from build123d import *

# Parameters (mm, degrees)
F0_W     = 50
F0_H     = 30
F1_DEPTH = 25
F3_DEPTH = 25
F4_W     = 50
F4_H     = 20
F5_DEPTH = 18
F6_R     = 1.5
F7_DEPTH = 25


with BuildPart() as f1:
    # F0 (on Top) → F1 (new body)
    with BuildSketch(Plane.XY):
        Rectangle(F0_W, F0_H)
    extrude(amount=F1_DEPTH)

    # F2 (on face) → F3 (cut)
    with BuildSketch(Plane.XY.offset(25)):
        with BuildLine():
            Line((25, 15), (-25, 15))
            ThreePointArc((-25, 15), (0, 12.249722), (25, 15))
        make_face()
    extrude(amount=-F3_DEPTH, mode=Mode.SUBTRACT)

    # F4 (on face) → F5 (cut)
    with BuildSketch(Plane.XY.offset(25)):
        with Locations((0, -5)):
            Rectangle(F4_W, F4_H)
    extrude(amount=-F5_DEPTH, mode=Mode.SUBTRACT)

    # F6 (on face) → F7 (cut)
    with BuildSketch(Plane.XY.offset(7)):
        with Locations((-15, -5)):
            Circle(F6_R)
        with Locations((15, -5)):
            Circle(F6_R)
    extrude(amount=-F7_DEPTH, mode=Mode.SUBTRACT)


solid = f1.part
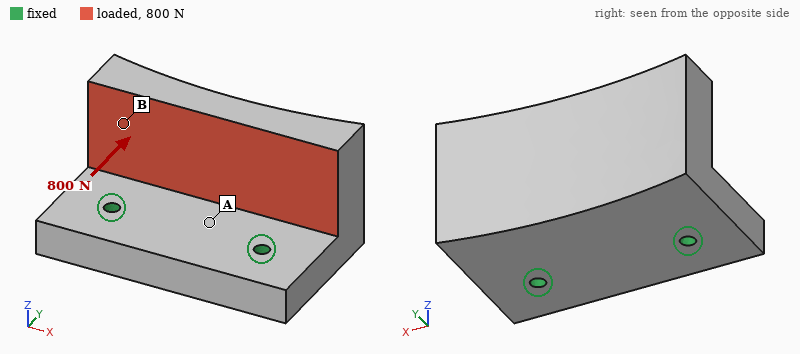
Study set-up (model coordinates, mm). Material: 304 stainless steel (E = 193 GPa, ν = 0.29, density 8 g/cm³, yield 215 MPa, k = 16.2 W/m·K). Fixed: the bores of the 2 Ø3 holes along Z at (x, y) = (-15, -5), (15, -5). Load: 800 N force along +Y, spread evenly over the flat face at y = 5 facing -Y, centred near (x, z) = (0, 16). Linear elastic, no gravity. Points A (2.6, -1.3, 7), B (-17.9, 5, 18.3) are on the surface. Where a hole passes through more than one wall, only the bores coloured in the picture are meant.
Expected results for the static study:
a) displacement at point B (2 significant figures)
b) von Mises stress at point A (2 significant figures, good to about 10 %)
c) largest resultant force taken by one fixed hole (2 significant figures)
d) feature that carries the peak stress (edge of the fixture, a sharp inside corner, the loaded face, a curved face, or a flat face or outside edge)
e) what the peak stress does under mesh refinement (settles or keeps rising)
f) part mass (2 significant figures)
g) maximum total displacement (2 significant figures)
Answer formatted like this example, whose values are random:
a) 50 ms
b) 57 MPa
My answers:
a) 10 µm
b) 16 MPa
c) 400 N
d) edge of the fixture
e) keeps rising
f) 140 g
g) 17 µm
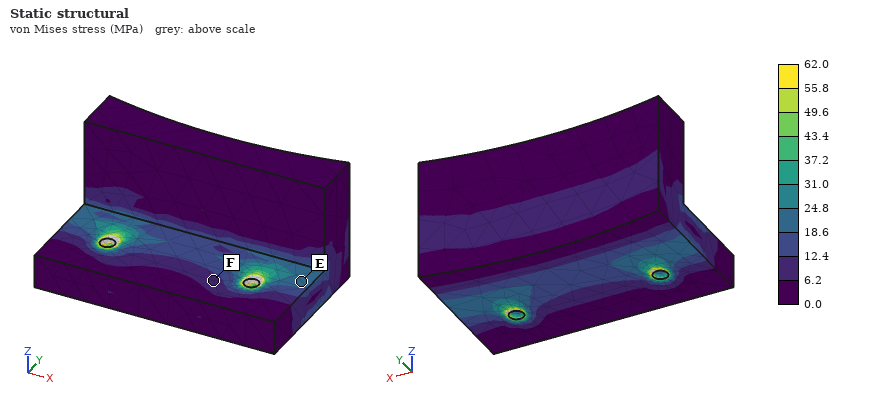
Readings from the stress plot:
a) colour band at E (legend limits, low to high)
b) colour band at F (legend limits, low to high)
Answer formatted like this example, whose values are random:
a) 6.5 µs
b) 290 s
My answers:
a) 18.6 to 24.8 MPa
b) 6.2 to 12.4 MPa
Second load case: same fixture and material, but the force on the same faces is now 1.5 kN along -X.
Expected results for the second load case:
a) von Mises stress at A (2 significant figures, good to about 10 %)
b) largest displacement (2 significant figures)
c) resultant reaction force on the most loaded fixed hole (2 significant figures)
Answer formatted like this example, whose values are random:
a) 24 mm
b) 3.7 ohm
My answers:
a) 18 MPa
b) 9.7 µm
c) 1.0 kN
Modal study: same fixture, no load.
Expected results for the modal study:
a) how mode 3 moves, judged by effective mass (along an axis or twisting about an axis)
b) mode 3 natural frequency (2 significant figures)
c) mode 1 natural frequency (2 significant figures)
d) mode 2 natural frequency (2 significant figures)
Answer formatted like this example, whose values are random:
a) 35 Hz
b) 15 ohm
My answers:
a) along X
b) 13 kHz
c) 4600 Hz
d) 8000 Hz
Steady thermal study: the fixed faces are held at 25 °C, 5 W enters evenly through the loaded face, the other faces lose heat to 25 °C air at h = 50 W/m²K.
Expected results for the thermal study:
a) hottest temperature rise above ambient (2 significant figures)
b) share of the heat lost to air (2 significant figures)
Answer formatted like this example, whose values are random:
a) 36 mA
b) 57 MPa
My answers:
a) 16 K
b) 40 %
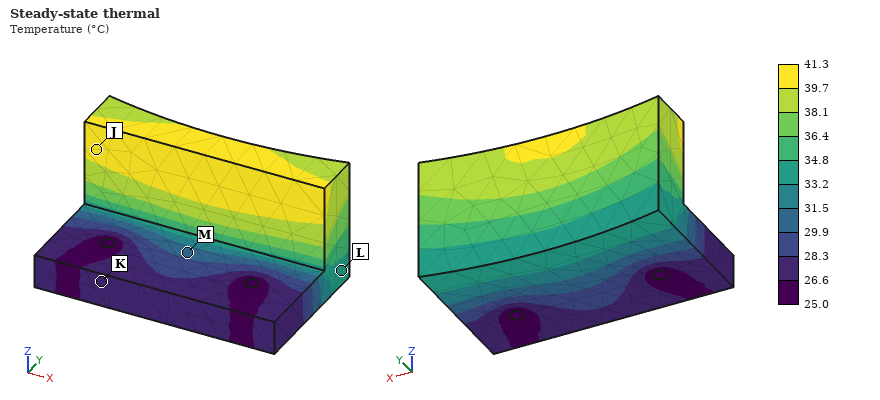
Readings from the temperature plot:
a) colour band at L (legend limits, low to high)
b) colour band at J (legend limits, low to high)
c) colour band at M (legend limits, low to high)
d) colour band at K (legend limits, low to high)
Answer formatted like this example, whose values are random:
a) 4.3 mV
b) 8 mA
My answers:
a) 33.2 to 34.8 °C
b) 39.7 to 41.3 °C
c) 29.9 to 31.5 °C
d) 26.6 to 28.3 °C
